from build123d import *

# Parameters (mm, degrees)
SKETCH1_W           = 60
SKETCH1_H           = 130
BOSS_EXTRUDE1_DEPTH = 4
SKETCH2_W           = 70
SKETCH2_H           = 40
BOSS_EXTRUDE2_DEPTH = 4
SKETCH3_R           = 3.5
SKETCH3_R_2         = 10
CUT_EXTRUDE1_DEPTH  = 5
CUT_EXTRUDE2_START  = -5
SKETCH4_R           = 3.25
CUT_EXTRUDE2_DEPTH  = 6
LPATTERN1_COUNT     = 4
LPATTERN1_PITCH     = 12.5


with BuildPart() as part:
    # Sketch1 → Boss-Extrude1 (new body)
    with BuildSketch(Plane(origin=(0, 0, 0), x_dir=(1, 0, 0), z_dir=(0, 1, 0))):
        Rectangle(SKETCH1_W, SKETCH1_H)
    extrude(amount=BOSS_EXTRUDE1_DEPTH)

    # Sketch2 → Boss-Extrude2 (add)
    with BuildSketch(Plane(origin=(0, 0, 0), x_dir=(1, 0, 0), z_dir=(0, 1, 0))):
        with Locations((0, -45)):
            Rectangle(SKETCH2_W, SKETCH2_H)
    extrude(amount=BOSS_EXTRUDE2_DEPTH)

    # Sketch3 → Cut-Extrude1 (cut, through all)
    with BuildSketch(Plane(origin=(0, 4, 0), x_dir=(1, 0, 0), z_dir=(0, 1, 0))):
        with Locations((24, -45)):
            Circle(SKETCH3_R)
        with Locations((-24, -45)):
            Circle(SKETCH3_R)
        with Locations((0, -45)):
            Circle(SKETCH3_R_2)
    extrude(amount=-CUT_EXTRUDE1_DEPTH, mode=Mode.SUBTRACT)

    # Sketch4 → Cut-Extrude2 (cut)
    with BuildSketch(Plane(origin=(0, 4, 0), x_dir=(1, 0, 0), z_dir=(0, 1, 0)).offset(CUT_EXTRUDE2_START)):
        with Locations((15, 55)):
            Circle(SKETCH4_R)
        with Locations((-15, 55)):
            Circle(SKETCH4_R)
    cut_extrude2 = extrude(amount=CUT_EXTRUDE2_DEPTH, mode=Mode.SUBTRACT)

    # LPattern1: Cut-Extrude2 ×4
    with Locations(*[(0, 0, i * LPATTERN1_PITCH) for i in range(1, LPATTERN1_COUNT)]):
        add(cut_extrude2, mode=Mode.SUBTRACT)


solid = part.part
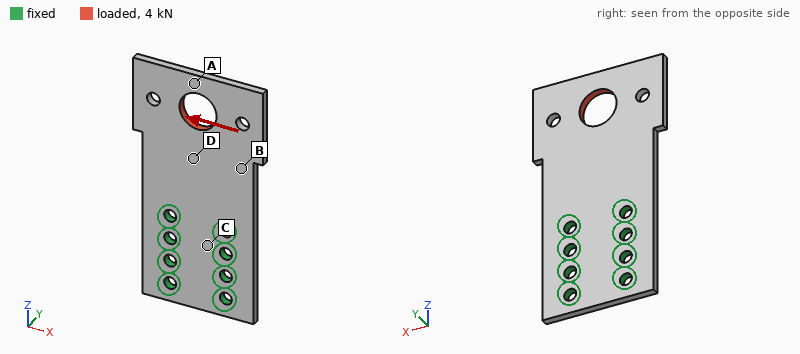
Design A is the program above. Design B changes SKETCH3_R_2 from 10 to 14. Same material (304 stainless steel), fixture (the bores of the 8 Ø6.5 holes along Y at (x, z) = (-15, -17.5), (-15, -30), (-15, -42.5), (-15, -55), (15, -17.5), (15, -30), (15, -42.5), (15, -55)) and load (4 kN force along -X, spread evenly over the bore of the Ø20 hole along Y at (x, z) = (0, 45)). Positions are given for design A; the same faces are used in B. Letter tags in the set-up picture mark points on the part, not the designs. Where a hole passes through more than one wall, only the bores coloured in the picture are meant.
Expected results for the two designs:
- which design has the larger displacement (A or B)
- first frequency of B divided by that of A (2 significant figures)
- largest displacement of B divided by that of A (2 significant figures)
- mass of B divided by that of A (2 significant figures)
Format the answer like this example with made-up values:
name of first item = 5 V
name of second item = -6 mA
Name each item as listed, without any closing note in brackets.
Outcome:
which design has the larger displacement = B
first frequency of B divided by that of A = 1.1
largest displacement of B divided by that of A = 1.2
mass of B divided by that of A = 0.96
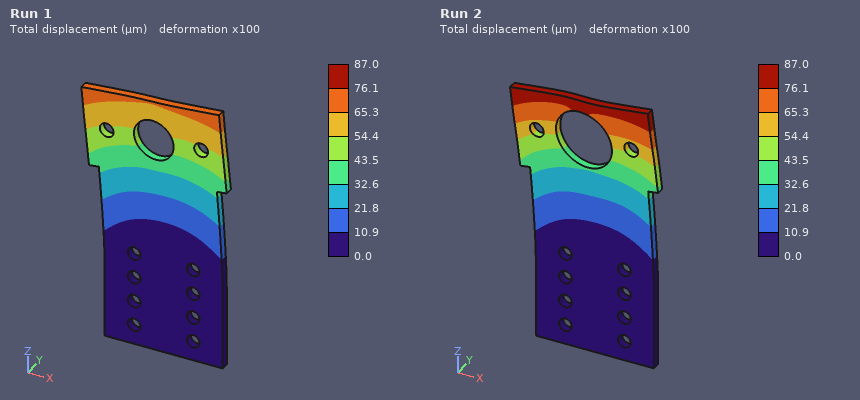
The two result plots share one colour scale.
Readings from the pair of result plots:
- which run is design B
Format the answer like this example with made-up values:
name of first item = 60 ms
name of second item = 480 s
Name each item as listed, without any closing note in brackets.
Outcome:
which run is design B = Run 2
